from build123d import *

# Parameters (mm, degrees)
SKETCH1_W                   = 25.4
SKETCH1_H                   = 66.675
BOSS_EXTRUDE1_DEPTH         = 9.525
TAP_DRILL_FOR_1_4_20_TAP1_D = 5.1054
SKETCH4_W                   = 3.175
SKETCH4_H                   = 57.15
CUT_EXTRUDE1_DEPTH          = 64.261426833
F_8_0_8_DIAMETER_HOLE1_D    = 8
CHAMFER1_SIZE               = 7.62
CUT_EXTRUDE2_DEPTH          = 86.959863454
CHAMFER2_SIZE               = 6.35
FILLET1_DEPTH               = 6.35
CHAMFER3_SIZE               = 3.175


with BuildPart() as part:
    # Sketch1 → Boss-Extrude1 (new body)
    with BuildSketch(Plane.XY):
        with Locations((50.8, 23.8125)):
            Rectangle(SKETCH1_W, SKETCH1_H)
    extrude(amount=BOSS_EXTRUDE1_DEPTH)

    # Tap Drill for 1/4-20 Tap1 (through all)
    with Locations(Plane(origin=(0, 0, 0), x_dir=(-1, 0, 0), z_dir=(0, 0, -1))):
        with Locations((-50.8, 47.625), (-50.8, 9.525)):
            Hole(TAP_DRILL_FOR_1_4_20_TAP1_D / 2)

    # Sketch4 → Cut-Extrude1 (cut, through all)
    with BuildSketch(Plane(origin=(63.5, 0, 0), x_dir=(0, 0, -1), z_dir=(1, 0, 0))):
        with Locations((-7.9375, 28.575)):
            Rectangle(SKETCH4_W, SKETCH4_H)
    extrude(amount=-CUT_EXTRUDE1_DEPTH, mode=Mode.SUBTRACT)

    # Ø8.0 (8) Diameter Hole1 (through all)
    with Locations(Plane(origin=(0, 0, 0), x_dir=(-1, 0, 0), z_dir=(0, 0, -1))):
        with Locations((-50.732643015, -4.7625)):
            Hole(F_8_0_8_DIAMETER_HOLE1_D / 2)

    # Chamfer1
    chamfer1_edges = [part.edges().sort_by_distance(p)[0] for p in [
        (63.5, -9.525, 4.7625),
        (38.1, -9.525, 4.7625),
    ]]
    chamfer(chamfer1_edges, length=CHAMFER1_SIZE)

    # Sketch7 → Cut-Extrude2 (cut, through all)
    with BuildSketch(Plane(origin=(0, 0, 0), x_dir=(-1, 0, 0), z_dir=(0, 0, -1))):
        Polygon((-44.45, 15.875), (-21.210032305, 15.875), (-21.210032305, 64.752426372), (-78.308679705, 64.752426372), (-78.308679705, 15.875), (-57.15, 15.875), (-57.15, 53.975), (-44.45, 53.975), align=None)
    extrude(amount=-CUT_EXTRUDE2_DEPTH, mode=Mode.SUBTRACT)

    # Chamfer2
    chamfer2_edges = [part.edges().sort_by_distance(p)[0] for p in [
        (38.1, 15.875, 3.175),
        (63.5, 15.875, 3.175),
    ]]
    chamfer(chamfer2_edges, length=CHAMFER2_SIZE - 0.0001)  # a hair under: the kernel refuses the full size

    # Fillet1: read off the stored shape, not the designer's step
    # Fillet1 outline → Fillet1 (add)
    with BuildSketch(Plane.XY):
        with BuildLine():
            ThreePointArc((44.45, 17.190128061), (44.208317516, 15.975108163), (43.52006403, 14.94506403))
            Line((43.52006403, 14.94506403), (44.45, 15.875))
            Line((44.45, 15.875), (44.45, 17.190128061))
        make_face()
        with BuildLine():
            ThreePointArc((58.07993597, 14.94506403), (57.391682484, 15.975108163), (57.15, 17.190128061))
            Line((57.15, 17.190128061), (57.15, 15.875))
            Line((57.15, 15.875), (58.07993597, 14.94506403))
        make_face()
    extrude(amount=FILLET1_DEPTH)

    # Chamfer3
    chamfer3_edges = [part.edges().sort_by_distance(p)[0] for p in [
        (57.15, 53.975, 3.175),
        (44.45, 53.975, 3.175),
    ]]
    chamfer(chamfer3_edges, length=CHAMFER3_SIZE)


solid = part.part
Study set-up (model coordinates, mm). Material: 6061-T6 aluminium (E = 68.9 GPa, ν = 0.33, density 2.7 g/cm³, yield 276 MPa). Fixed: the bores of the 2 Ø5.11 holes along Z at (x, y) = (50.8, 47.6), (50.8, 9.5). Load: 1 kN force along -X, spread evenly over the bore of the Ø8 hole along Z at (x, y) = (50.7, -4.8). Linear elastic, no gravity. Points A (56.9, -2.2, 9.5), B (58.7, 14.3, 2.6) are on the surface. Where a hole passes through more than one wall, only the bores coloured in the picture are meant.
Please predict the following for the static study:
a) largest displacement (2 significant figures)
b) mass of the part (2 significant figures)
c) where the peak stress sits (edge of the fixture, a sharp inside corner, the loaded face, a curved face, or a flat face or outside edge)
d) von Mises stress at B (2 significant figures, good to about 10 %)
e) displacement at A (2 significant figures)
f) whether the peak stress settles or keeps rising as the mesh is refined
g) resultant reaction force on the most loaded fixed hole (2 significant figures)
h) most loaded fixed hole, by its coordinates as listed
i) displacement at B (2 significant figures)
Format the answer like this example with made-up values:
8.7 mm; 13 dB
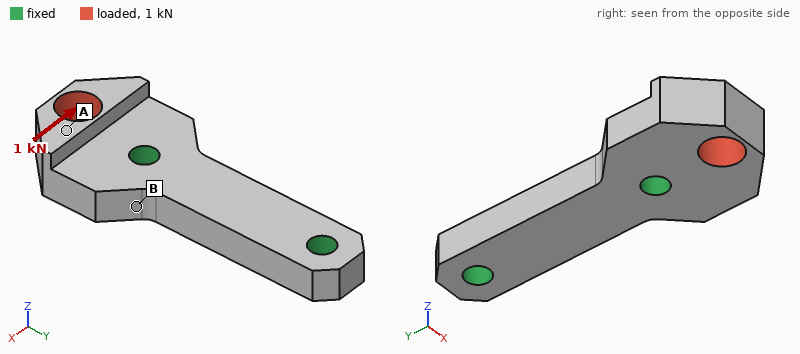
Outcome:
25 µm; 17 g; edge of the fixture; 27 MPa; 15 µm; keeps rising; 1.2 kN; (50.8, 9.5); 5.1 µm
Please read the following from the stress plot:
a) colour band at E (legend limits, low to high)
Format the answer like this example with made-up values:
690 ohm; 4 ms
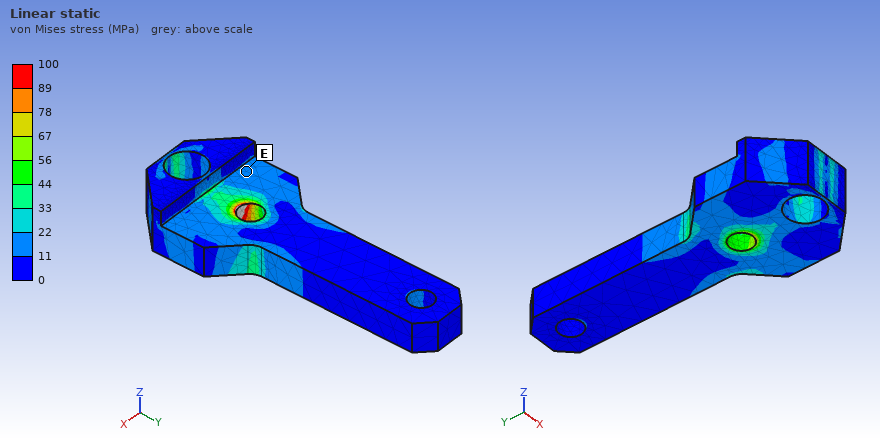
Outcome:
11 to 22 MPa
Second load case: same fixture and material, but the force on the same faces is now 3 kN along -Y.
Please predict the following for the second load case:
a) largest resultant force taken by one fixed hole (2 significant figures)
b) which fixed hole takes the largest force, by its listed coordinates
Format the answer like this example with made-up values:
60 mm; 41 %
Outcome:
2.8 kN; (50.8, 9.5)
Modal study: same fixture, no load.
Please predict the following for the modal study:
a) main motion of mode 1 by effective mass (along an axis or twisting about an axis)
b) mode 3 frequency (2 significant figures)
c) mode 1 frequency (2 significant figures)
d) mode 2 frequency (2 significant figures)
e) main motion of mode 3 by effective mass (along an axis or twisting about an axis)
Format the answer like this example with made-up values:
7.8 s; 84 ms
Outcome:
along Z; 19 kHz; 14 kHz; 17 kHz; twisting about Y
